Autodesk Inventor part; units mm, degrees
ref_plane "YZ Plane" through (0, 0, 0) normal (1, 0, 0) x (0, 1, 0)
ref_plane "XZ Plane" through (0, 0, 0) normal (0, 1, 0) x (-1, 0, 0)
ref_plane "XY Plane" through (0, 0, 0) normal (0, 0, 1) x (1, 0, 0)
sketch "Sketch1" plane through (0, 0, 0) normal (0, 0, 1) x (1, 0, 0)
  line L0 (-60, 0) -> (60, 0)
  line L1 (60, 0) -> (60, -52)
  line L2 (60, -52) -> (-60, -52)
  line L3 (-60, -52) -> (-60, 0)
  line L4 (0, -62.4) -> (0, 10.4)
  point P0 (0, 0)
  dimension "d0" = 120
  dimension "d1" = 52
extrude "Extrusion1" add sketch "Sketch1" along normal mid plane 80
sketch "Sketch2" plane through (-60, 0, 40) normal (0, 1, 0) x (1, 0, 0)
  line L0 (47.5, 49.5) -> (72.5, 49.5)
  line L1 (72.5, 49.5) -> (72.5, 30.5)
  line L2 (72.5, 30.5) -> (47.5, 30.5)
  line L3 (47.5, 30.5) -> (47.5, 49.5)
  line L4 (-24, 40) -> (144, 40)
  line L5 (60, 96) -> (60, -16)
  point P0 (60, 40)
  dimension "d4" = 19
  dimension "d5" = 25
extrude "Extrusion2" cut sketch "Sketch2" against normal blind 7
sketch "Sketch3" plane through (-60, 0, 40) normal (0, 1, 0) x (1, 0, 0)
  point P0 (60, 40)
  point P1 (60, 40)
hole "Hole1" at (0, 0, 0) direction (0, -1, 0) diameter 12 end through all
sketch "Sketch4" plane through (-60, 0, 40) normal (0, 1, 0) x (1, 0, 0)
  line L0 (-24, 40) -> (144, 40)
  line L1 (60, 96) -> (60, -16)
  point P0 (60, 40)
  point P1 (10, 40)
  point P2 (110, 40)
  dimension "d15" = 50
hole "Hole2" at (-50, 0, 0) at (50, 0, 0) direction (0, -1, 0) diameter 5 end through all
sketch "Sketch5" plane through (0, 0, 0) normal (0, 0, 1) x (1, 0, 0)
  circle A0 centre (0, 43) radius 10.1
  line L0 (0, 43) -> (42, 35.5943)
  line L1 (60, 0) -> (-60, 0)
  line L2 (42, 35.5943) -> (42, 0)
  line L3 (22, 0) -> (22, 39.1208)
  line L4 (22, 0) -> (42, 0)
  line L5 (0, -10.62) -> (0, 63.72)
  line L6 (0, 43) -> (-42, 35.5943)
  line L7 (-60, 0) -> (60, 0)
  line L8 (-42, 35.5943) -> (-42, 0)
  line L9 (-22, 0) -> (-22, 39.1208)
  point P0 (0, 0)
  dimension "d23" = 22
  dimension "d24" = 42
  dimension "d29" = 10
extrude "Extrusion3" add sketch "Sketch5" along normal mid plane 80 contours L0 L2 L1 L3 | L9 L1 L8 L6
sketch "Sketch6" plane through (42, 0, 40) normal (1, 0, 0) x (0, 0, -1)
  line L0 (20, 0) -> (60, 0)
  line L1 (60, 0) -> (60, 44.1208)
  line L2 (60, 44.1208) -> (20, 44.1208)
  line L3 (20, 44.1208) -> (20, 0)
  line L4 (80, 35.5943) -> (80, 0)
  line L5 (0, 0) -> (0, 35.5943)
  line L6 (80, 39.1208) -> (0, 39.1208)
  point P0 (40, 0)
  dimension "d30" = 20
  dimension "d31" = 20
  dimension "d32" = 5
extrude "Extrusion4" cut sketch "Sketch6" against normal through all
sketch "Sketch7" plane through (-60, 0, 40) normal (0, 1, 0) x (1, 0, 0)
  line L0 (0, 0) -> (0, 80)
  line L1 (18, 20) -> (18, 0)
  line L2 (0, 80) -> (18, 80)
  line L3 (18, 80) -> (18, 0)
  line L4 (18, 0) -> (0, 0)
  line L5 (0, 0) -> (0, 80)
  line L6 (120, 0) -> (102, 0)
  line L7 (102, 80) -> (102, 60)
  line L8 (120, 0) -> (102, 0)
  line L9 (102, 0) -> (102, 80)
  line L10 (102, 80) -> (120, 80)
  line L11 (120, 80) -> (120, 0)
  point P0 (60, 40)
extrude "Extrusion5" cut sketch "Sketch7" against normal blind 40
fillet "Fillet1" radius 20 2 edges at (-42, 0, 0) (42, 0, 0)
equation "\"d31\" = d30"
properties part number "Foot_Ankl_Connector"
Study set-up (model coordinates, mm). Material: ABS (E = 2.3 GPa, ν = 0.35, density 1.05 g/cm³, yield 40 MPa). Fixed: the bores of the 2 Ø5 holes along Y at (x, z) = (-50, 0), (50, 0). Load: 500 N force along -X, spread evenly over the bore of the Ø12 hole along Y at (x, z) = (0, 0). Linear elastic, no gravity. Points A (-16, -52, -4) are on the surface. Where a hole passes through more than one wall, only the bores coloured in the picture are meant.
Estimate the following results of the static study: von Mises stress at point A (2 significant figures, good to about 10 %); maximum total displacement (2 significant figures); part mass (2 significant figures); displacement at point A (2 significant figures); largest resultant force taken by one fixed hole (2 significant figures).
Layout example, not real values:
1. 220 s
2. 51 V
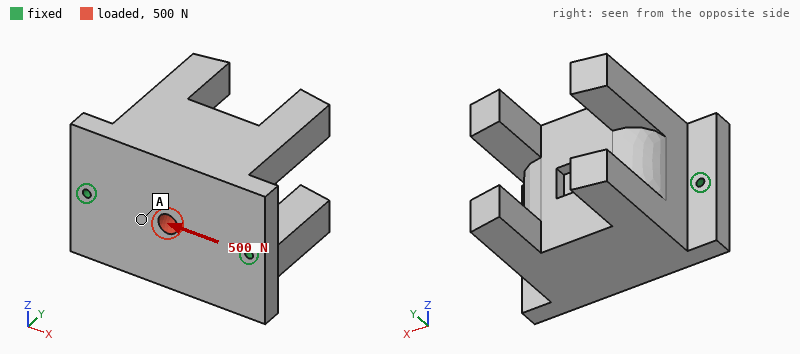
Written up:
1. 0.29 MPa
2. 19 µm
3. 450 g
4. 8.1 µm
5. 260 N
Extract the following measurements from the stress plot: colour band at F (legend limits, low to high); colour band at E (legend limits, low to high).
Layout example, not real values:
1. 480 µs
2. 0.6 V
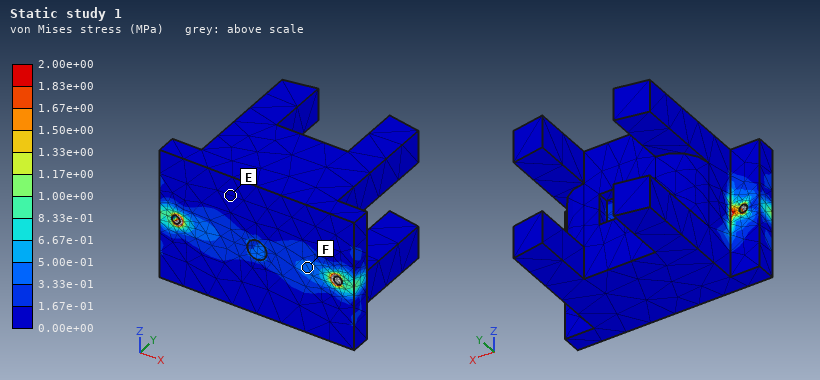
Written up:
1. 3.33e-01 to 5.00e-01 MPa
2. 0.00e+00 to 1.67e-01 MPa
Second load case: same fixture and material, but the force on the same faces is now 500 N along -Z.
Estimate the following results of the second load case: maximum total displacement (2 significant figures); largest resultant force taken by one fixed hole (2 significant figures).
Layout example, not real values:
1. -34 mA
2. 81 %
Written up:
1. 0.36 mm
2. 250 N
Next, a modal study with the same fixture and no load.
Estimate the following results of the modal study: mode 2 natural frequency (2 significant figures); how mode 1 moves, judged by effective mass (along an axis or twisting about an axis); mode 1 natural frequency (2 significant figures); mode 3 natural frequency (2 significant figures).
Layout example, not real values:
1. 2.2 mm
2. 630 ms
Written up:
1. 1100 Hz
2. along Z
3. 270 Hz
4. 1100 Hz
